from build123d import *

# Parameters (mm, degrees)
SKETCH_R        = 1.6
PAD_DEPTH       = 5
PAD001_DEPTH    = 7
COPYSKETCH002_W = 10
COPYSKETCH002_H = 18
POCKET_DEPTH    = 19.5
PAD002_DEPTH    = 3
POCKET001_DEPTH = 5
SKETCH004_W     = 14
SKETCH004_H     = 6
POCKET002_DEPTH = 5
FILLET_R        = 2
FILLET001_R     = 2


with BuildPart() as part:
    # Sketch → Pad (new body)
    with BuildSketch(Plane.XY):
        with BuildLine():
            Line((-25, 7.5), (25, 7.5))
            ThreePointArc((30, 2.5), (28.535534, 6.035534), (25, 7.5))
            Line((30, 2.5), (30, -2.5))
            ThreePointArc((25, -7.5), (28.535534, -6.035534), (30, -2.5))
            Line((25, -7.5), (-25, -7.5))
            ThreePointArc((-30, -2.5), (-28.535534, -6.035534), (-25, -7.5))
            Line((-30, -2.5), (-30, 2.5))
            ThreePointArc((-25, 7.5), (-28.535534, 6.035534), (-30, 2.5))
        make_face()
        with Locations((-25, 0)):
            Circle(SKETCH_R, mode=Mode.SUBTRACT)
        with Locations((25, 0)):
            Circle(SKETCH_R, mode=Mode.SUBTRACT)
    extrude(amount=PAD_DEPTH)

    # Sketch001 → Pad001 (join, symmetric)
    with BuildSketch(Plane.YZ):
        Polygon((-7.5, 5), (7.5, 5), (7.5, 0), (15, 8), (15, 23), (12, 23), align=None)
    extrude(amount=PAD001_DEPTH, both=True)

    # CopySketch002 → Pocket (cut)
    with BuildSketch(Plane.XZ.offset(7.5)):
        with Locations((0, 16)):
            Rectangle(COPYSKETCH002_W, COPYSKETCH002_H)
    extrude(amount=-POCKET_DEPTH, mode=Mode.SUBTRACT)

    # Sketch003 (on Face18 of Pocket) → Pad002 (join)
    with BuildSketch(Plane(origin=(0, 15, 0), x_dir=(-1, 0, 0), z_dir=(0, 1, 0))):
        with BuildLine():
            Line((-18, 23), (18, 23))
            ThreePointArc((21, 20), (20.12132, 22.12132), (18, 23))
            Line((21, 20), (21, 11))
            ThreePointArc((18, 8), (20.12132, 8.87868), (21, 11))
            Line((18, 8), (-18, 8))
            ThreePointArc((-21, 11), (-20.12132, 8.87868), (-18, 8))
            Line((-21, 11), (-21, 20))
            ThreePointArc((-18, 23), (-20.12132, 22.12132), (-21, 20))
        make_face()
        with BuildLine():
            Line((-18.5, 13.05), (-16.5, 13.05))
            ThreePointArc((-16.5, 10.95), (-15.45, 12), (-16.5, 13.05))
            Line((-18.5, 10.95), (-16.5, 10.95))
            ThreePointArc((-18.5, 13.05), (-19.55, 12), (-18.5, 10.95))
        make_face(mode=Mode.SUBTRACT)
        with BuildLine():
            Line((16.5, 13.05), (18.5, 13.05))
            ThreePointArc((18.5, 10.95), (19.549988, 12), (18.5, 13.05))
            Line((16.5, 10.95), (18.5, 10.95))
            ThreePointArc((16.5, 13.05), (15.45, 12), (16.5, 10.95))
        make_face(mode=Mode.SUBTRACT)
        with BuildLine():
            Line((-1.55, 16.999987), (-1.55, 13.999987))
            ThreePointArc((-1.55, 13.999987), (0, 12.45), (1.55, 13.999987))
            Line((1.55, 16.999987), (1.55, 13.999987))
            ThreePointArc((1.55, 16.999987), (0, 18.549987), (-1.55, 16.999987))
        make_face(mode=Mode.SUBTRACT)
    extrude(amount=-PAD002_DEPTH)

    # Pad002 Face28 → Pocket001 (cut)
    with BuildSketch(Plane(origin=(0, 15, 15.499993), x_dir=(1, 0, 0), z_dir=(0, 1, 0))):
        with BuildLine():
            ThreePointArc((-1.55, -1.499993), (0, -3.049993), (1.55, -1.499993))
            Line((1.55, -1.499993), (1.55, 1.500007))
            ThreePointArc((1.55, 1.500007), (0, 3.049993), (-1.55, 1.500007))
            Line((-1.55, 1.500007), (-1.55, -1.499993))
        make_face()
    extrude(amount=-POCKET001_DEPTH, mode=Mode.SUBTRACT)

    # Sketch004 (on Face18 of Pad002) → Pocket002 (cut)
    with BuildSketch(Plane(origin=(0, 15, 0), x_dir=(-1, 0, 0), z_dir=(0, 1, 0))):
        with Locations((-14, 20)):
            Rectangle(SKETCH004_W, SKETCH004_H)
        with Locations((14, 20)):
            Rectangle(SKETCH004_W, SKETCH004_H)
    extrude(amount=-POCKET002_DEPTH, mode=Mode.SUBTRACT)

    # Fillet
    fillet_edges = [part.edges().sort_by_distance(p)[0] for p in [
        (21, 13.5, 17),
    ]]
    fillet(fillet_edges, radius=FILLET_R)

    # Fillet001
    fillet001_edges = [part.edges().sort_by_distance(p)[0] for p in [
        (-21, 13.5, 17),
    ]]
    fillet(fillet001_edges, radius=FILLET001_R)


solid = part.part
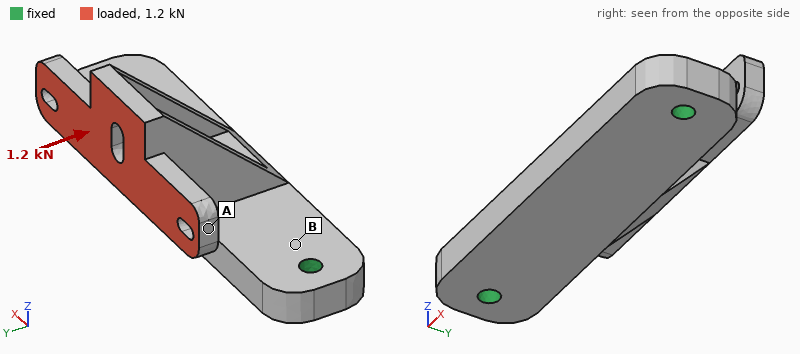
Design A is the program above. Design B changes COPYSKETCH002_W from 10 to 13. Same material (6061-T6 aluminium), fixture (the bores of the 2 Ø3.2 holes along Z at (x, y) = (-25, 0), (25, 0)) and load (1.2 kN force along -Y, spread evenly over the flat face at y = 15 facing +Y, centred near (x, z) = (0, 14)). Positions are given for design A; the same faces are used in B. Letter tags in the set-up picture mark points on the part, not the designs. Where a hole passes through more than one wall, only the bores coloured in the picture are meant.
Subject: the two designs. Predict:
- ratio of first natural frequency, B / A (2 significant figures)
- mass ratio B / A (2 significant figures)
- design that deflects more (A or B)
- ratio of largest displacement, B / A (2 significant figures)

1.0
0.94
B
1.2
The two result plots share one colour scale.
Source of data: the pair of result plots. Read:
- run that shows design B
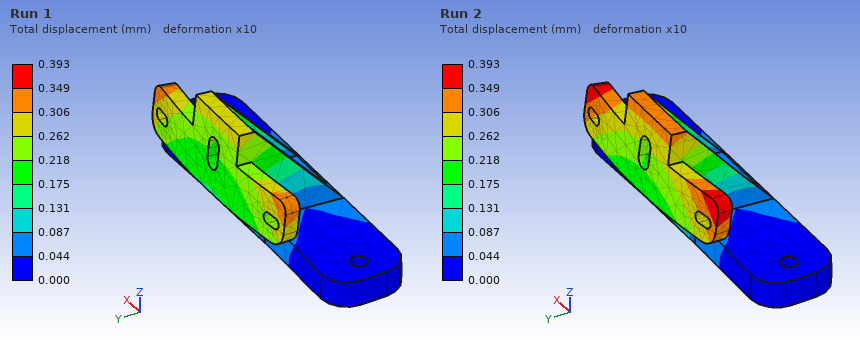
Run 2
